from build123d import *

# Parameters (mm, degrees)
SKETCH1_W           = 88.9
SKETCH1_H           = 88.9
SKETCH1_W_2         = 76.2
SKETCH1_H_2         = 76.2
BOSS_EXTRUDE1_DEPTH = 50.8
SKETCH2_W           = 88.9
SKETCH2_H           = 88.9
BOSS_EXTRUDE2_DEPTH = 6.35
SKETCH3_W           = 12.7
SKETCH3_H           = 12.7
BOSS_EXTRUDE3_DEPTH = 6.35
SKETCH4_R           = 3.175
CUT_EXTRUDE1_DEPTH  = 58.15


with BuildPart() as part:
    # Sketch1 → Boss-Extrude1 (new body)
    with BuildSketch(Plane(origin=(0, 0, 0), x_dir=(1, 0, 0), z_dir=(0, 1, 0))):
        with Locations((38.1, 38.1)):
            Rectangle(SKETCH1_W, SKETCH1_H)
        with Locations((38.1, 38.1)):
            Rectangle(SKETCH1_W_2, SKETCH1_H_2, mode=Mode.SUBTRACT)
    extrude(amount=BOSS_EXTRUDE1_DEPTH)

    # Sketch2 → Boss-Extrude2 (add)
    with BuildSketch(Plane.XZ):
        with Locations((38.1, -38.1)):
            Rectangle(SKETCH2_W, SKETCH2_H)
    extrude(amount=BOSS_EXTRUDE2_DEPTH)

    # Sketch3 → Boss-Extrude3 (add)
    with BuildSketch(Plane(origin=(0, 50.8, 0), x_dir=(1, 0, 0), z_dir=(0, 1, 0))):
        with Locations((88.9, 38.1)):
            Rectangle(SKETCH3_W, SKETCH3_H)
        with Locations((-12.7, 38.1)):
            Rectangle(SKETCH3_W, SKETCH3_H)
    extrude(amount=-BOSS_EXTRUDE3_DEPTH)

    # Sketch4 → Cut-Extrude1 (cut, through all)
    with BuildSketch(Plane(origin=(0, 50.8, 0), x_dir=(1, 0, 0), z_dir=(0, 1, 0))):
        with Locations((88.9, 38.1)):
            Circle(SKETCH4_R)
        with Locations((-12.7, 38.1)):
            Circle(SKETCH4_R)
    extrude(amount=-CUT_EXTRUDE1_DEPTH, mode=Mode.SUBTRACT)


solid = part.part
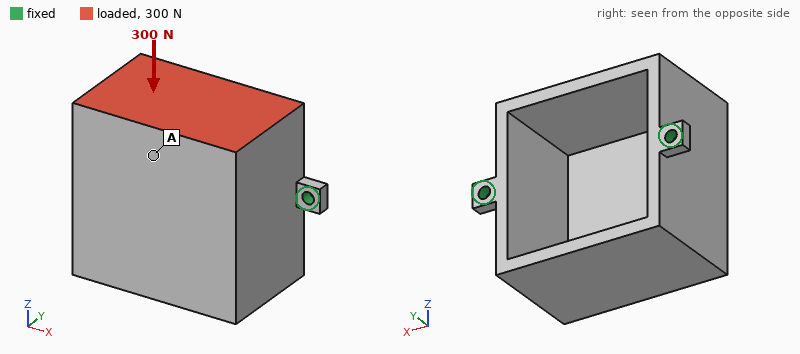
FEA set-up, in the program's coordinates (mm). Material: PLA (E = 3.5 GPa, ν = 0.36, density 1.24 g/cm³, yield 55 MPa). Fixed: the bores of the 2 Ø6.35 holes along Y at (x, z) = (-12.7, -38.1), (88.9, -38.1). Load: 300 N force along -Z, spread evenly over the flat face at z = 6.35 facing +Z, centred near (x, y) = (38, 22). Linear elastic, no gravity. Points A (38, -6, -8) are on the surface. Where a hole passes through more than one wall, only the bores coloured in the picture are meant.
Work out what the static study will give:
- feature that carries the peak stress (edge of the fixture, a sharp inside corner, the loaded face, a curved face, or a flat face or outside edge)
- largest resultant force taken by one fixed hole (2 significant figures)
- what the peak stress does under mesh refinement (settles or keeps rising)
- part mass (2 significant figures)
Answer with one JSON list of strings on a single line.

["edge of the fixture", "150 N", "keeps rising", "200 g"]
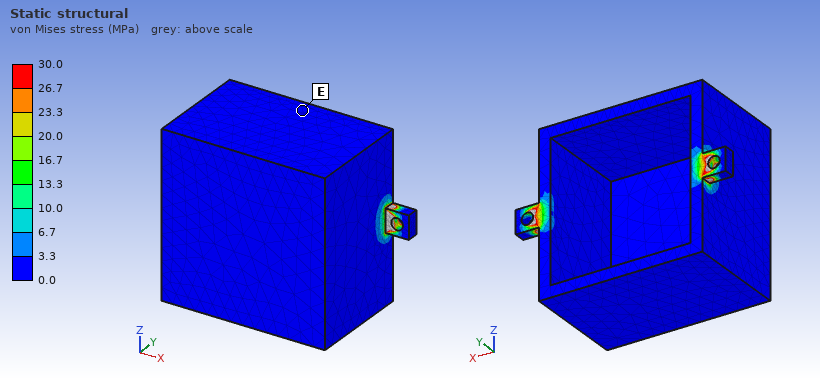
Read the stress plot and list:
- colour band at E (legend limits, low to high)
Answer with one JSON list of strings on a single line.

["0.0 to 3.3 MPa"]
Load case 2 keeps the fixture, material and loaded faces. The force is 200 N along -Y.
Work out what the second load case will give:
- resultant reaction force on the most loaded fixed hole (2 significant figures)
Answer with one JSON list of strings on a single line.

["100 N"]
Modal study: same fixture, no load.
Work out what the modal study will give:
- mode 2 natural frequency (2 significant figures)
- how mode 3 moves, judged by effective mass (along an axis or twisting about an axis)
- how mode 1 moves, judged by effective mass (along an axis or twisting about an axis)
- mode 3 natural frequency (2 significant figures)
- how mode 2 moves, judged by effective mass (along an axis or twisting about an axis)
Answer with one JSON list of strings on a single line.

["440 Hz", "twisting about Y", "along Z", "470 Hz", "along X"]
